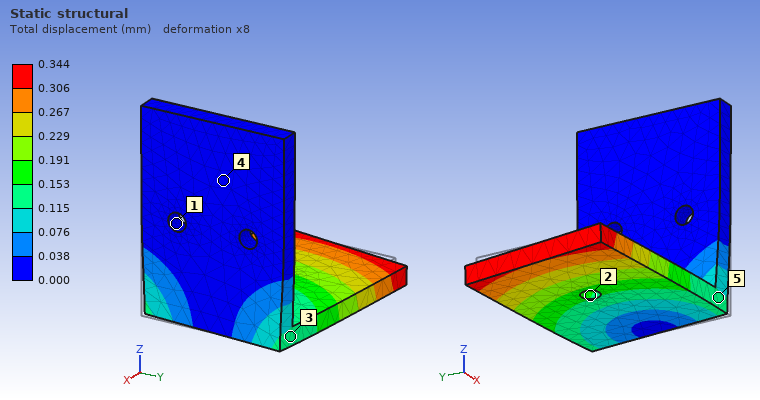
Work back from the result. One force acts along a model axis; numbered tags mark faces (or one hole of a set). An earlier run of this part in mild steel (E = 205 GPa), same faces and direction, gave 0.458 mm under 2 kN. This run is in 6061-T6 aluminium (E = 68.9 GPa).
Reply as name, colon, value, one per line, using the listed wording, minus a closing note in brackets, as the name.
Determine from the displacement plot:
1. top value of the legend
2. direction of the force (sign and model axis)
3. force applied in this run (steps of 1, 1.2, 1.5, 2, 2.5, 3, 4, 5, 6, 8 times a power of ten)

top value of the legend: 0.344 mm
direction of the force: +Y
force applied in this run: 500 N
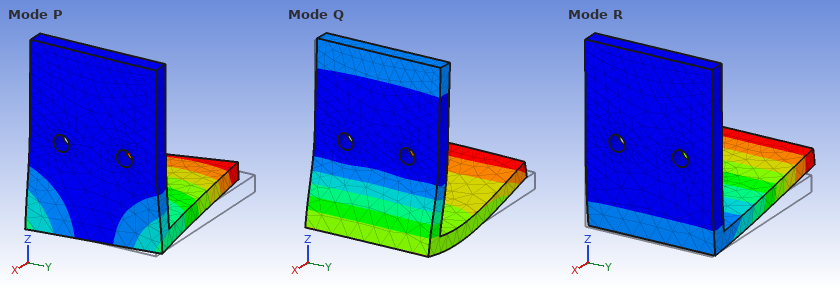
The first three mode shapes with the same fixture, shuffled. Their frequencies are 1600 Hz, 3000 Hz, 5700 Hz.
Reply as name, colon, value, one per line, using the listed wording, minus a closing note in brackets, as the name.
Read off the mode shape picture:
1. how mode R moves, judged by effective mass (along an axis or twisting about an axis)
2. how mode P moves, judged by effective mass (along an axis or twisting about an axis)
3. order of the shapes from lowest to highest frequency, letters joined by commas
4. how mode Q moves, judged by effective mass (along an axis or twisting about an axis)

how mode R moves, judged by effective mass: along Z
how mode P moves, judged by effective mass: along Y
order of the shapes from lowest to highest frequency, letters joined by commas: R, P, Q
how mode Q moves, judged by effective mass: along X
